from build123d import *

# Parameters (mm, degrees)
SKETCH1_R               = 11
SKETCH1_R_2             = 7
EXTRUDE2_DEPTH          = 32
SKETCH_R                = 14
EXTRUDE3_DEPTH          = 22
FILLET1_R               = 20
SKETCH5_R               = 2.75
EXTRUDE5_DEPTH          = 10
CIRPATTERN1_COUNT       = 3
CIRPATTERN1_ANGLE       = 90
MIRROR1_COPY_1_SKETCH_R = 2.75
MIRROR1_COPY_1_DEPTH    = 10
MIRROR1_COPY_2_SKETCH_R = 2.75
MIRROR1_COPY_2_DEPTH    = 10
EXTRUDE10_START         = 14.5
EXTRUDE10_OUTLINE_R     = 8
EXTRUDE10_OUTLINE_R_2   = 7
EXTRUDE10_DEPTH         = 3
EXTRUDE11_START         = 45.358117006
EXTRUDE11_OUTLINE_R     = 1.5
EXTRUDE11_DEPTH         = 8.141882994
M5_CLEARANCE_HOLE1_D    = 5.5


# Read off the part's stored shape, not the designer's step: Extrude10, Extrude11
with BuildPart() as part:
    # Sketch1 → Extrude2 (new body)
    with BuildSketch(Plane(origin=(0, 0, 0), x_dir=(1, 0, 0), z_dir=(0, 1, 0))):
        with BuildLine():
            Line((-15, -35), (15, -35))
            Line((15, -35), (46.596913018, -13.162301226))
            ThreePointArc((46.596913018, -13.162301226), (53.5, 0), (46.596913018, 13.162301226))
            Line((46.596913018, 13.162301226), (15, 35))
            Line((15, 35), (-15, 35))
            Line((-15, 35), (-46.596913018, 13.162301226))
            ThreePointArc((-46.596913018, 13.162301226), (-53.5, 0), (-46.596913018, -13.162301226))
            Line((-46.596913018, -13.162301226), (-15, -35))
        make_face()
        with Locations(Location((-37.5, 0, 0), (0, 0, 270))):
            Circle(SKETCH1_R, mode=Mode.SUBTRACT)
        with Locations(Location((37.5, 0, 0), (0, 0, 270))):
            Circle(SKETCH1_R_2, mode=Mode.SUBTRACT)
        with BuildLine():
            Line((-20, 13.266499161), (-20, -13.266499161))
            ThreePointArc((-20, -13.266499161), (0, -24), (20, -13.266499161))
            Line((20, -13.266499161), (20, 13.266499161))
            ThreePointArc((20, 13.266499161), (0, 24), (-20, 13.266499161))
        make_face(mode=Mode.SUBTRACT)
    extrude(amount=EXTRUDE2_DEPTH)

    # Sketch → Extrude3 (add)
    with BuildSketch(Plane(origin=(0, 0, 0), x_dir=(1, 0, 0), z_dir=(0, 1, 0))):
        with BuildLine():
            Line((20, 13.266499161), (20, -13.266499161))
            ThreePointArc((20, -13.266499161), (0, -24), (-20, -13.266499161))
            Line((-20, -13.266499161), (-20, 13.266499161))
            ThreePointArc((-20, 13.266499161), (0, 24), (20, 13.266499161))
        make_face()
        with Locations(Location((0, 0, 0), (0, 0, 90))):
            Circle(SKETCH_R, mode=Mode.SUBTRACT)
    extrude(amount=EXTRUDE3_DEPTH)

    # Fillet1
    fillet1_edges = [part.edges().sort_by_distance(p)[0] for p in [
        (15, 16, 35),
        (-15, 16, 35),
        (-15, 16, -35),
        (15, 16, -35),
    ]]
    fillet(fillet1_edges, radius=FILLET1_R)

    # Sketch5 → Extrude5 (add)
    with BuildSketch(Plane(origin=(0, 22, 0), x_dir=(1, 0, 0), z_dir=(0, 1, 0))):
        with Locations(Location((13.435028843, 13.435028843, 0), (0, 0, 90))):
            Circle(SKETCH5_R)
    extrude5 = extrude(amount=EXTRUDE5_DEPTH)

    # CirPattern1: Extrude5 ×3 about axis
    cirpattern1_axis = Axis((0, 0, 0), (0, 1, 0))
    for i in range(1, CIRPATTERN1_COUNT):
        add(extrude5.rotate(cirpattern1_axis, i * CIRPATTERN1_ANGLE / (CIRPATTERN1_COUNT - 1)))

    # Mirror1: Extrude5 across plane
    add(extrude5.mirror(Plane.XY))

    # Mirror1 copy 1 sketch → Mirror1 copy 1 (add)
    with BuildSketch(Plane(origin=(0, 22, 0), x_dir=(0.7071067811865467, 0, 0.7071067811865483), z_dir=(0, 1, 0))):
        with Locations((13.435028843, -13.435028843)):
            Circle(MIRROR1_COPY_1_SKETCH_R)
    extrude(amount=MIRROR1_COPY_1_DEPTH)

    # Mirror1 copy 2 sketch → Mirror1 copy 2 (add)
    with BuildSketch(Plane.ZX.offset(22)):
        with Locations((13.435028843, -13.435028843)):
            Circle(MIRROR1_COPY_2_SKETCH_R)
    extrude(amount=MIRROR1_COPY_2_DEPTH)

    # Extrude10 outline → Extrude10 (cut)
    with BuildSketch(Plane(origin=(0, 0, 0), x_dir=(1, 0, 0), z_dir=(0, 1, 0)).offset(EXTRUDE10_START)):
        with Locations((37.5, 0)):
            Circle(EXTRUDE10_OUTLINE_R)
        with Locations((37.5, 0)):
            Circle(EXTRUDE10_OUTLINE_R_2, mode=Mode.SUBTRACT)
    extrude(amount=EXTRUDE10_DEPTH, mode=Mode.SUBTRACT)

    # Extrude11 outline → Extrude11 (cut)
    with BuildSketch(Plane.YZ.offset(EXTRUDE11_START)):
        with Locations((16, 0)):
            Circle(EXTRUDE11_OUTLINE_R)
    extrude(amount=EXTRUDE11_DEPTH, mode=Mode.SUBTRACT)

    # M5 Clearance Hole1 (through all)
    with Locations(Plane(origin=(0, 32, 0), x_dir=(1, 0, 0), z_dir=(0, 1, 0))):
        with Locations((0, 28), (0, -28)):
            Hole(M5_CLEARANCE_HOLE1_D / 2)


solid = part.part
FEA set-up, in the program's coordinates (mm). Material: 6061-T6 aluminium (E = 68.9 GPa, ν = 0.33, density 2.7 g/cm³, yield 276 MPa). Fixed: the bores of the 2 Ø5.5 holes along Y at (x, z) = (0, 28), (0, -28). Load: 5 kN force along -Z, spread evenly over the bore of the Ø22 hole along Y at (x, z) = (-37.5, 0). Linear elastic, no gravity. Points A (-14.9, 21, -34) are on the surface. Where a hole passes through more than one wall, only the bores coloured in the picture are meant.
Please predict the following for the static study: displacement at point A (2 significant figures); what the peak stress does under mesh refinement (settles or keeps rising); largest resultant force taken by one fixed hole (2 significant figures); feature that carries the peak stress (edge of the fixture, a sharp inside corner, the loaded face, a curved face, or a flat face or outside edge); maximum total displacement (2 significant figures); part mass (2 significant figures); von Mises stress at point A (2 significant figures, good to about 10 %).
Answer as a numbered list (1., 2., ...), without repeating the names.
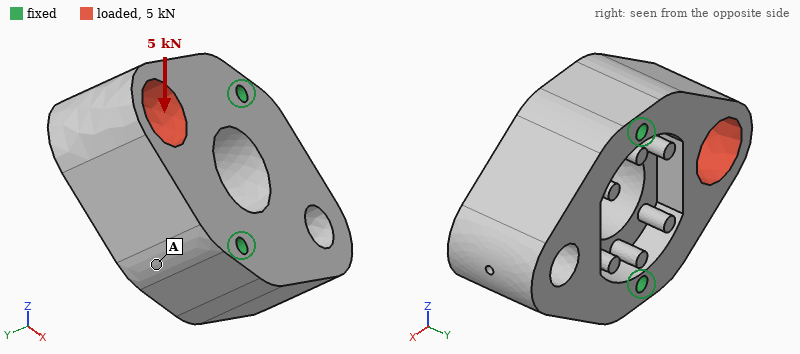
1. 4.8 µm
2. keeps rising
3. 3.9 kN
4. edge of the fixture
5. 20 µm
6. 340 g
7. 3.8 MPa
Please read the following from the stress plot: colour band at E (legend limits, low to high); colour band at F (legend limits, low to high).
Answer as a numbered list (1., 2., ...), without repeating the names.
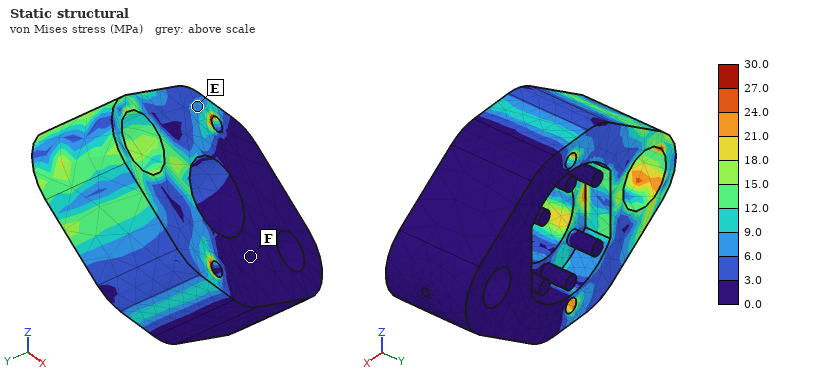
1. 6.0 to 9.0 MPa
2. 0.0 to 3.0 MPa
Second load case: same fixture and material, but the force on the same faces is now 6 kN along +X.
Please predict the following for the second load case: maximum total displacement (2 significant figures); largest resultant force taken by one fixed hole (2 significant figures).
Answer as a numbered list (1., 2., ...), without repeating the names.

1. 7.7 µm
2. 3.2 kN
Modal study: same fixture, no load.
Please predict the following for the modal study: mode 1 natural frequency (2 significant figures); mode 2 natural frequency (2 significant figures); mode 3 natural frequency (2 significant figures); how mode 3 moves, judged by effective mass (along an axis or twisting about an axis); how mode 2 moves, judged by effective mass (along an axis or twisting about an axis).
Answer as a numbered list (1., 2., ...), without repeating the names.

1. 7100 Hz
2. 8400 Hz
3. 12 kHz
4. twisting about Y
5. along Y
